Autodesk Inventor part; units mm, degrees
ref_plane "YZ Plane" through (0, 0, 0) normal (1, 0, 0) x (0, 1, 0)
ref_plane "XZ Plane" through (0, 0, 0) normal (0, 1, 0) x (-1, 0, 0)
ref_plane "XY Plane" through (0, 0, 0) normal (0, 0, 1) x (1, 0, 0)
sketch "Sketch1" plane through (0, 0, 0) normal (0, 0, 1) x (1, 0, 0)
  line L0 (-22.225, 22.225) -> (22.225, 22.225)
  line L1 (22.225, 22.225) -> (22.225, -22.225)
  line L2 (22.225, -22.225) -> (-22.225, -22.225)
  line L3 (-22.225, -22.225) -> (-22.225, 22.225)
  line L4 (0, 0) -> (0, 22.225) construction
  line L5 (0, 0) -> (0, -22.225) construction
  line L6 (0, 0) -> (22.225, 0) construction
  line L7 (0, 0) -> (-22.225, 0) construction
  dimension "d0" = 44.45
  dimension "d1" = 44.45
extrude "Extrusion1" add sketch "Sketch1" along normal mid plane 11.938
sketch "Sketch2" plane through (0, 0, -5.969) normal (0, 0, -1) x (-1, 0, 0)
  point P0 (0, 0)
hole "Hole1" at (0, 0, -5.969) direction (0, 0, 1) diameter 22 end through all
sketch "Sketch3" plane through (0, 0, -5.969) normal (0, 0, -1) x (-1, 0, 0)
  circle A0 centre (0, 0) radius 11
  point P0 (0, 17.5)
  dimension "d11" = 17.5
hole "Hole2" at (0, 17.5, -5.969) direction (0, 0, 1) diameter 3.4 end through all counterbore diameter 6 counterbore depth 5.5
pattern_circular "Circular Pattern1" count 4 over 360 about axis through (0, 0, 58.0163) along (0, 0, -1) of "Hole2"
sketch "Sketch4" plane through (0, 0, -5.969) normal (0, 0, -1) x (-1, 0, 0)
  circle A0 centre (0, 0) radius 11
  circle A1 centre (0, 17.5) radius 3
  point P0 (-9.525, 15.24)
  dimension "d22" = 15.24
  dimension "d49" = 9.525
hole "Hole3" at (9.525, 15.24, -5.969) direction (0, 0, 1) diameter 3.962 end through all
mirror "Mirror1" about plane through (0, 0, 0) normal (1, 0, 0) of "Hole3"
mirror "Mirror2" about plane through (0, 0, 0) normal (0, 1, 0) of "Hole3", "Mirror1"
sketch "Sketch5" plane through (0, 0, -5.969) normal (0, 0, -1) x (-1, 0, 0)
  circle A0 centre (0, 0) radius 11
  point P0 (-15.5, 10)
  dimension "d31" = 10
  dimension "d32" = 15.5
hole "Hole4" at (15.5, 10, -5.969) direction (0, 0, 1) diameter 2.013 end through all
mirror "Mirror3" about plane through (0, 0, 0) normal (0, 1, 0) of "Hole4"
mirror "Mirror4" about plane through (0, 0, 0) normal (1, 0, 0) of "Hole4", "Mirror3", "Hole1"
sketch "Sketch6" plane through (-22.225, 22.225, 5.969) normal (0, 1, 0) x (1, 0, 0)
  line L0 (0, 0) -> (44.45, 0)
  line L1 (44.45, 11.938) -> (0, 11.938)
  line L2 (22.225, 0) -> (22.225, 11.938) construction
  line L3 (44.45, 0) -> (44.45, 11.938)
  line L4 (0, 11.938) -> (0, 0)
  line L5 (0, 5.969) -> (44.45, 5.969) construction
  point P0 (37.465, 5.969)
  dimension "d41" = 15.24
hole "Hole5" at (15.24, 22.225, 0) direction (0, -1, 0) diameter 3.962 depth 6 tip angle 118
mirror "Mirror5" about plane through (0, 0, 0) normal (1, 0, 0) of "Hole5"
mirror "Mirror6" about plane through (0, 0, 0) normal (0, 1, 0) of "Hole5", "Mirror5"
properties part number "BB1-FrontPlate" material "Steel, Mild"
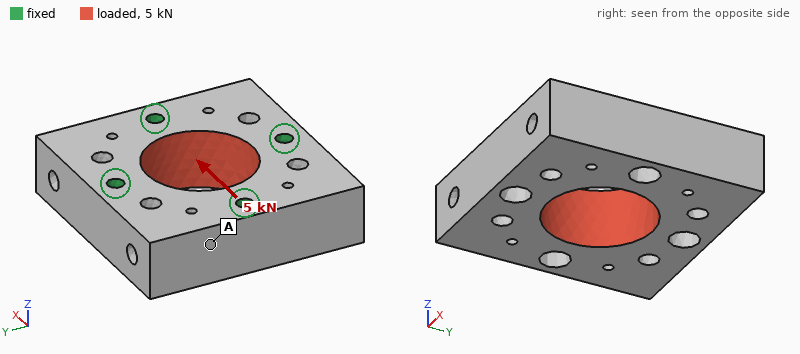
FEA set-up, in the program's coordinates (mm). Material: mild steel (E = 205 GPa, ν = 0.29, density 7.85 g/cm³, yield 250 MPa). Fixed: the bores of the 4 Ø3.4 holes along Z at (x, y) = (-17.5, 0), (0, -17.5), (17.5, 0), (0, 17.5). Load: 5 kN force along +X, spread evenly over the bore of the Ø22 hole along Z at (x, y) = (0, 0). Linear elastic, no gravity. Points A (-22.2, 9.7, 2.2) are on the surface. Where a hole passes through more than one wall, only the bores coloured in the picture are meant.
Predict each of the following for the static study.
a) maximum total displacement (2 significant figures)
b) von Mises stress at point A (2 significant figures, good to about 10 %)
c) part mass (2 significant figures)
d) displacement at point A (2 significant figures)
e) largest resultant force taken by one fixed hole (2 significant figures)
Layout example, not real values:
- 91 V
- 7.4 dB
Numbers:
- 1.3 µm
- 5.5 MPa
- 130 g
- 0.72 µm
- 1.3 kN
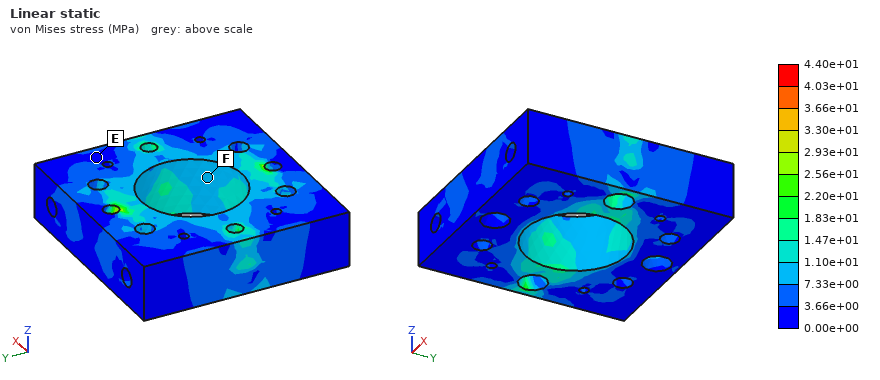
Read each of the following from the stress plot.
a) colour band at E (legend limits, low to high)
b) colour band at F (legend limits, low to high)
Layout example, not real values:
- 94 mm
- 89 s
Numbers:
- 0.00e+00 to 3.66e+00 MPa
- 7.33e+00 to 1.10e+01 MPa
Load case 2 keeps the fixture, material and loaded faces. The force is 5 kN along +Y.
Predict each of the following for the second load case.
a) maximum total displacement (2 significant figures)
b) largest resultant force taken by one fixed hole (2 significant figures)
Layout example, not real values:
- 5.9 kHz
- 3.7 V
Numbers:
- 1.3 µm
- 1.3 kN
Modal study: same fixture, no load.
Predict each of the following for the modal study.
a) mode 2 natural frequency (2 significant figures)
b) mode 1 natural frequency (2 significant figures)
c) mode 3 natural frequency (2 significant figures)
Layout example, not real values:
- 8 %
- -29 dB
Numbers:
- 20 kHz
- 17 kHz
- 20 kHz
